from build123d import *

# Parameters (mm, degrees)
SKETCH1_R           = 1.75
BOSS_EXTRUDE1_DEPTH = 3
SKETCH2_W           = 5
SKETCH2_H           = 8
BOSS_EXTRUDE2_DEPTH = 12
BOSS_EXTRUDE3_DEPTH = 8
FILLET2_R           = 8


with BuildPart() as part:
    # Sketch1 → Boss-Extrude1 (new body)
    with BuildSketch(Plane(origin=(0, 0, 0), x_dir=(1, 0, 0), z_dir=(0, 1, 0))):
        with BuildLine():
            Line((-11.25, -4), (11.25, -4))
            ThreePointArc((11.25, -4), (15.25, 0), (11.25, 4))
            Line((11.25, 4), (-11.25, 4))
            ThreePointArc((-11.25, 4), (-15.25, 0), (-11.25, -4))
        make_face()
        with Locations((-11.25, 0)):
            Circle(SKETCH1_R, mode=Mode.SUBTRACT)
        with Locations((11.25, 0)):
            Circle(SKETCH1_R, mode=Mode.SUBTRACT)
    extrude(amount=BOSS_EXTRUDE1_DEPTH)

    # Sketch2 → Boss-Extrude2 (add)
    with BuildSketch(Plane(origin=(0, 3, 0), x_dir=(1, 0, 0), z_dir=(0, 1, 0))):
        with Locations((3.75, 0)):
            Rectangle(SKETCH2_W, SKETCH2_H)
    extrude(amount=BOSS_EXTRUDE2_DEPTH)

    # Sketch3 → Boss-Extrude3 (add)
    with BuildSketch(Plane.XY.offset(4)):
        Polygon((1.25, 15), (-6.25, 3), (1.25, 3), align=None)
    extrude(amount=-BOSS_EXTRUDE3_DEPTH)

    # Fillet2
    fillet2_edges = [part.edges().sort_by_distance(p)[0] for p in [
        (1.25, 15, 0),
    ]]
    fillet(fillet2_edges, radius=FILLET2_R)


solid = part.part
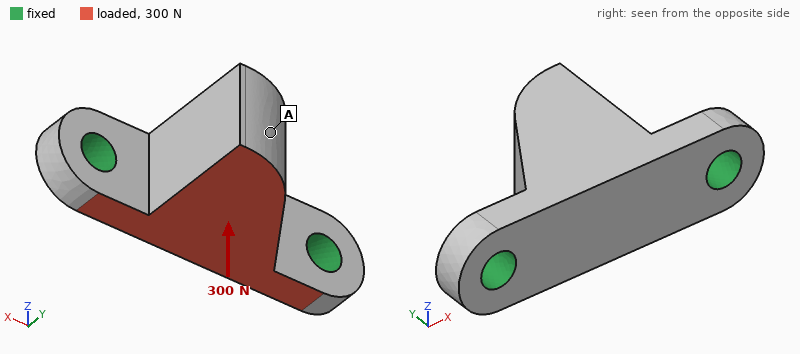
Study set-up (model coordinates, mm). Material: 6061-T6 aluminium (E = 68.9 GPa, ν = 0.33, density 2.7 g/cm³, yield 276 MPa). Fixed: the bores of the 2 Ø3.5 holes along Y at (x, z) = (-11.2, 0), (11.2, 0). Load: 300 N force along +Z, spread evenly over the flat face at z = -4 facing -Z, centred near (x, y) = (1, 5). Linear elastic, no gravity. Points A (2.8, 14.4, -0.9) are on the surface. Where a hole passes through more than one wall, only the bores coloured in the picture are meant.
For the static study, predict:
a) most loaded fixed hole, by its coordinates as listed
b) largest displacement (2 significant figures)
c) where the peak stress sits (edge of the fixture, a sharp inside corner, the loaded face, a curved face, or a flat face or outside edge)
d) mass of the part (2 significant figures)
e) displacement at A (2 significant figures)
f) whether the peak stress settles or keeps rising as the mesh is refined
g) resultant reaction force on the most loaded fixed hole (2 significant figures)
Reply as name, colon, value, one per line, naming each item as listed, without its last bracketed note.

most loaded fixed hole, by its coordinates as listed: (11.2, 0)
largest displacement: 27 µm
where the peak stress sits: edge of the fixture
mass of the part: 3.9 g
displacement at A: 25 µm
whether the peak stress settles or keeps rising as the mesh is refined: keeps rising
resultant reaction force on the most loaded fixed hole: 160 N
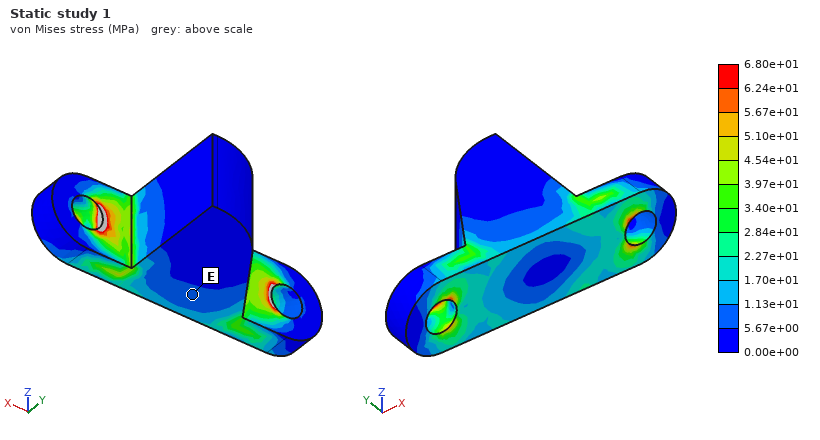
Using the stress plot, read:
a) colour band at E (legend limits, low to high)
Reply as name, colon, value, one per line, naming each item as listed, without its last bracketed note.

colour band at E: 5.67e+00 to 1.13e+01 MPa
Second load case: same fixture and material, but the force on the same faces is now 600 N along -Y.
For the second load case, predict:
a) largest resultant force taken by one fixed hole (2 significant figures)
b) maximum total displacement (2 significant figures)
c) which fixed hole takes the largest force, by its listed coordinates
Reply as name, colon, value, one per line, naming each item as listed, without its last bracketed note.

largest resultant force taken by one fixed hole: 360 N
maximum total displacement: 46 µm
which fixed hole takes the largest force, by its listed coordinates: (11.2, 0)
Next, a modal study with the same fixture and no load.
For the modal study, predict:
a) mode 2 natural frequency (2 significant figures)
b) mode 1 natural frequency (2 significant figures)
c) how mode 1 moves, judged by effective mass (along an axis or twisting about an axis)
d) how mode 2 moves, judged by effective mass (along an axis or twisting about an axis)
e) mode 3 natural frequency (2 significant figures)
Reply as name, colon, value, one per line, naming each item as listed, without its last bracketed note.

mode 2 natural frequency: 26 kHz
mode 1 natural frequency: 11 kHz
how mode 1 moves, judged by effective mass: along Z
how mode 2 moves, judged by effective mass: along Y
mode 3 natural frequency: 29 kHz
